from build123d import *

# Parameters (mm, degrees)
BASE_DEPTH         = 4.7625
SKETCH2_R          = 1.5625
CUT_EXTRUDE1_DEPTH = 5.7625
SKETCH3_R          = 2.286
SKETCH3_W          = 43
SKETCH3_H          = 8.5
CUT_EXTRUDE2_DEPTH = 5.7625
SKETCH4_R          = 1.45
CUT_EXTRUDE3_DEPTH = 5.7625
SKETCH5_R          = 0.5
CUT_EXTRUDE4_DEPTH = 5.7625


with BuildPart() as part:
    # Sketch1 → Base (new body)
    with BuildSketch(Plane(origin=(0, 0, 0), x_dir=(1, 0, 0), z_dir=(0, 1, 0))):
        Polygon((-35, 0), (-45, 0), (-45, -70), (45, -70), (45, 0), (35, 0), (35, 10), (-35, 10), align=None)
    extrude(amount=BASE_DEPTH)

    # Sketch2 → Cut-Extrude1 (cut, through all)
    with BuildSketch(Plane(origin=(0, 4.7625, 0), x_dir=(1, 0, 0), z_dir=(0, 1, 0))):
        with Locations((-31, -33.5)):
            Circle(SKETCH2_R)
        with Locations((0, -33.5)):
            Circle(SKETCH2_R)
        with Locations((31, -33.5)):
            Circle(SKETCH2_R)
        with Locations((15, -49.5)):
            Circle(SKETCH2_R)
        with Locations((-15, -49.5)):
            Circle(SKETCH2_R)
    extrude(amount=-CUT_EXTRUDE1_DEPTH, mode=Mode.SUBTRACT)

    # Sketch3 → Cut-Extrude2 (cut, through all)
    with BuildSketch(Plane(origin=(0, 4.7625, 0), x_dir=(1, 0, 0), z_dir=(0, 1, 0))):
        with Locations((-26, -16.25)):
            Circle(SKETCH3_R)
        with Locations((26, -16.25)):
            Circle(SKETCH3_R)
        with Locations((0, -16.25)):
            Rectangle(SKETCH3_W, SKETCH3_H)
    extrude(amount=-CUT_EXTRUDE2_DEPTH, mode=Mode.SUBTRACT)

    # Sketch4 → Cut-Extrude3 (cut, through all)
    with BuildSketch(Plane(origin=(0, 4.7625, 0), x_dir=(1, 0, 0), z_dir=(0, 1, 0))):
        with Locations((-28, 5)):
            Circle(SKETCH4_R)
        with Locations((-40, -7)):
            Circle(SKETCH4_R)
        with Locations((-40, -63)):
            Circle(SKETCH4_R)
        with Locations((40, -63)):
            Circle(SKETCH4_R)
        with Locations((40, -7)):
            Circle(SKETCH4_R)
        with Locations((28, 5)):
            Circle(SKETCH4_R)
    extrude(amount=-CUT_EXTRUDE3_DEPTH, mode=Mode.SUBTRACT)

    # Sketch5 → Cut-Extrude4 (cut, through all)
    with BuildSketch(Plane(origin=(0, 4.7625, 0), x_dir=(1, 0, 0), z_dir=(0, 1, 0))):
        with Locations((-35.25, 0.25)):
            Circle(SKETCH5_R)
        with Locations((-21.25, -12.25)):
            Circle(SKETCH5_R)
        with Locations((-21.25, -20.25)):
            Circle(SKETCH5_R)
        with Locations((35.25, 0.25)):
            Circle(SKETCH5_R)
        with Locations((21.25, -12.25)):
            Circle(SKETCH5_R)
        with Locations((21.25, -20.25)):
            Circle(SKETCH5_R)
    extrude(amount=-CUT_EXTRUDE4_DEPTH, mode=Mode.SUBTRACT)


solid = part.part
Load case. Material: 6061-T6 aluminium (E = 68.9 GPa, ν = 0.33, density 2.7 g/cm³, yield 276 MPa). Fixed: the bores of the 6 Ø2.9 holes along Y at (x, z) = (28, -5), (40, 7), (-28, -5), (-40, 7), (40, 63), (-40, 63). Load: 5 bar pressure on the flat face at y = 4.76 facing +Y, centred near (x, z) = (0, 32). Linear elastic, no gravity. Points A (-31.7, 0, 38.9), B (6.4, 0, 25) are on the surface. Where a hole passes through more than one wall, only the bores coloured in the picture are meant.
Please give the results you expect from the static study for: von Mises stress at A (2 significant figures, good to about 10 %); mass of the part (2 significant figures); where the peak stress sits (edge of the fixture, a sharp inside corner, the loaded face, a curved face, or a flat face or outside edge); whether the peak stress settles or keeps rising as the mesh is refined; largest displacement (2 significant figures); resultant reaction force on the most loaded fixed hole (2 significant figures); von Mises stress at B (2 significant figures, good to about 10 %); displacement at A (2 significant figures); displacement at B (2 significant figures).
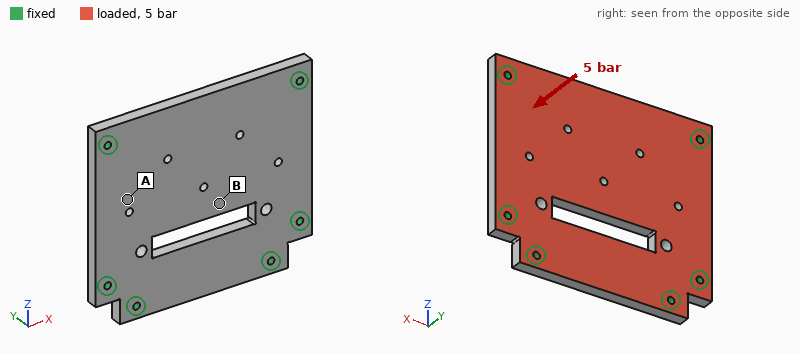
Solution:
22 MPa
84 g
edge of the fixture
keeps rising
0.15 mm
750 N
41 MPa
0.065 mm
0.14 mm
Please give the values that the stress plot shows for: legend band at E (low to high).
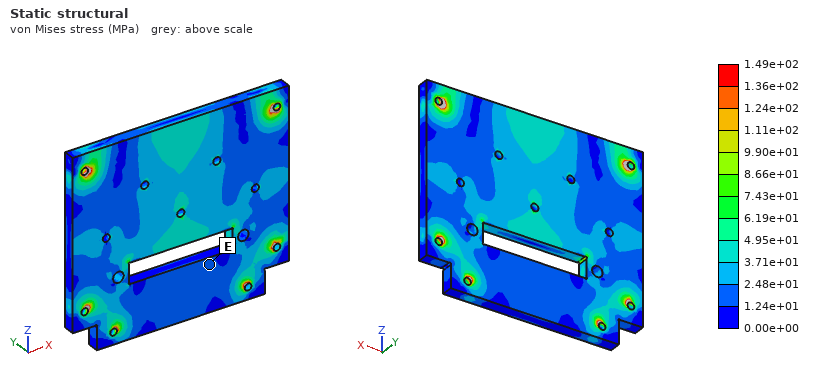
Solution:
1.24e+01 to 2.48e+01 MPa
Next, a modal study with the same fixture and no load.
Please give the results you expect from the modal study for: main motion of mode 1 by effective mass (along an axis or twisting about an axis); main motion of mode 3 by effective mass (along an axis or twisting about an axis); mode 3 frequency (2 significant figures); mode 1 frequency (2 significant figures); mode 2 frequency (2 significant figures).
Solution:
along Y
twisting about Z
6700 Hz
3100 Hz
5200 Hz
